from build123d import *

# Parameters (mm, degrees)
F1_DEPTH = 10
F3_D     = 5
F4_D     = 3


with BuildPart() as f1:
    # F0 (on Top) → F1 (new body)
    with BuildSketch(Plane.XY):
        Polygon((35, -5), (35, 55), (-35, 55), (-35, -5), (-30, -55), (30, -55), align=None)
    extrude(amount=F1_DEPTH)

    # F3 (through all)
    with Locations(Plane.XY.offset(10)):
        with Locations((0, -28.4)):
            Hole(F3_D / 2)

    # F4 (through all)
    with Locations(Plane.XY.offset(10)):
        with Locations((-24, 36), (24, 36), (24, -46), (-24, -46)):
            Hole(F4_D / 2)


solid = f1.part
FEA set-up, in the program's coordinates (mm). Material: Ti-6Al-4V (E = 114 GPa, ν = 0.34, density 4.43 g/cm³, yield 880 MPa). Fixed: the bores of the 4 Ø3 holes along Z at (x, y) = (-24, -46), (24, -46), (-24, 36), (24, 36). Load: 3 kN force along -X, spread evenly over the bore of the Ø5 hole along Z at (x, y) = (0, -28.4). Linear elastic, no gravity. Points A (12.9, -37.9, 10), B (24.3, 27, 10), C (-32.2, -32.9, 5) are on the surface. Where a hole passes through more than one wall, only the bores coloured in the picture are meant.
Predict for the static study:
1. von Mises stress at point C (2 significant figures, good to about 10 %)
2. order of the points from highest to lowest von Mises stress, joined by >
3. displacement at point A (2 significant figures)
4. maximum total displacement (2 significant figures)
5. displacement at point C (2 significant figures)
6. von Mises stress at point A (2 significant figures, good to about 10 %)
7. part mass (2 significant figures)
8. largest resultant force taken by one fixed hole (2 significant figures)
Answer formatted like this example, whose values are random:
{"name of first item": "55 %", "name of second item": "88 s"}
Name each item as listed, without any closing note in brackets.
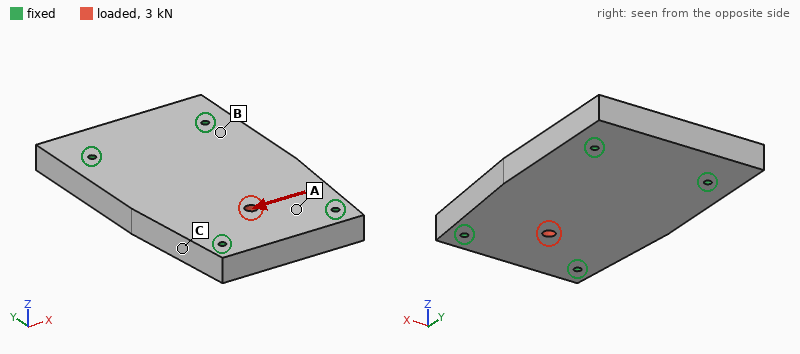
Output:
{"von Mises stress at point C": "4.9 MPa", "order of the points from highest to lowest von Mises stress, joined by >": "A > C > B", "displacement at point A": "1.3 µm", "maximum total displacement": "3.3 µm", "displacement at point C": "1.5 µm", "von Mises stress at point A": "8.8 MPa", "part mass": "330 g", "largest resultant force taken by one fixed hole": "1.2 kN"}
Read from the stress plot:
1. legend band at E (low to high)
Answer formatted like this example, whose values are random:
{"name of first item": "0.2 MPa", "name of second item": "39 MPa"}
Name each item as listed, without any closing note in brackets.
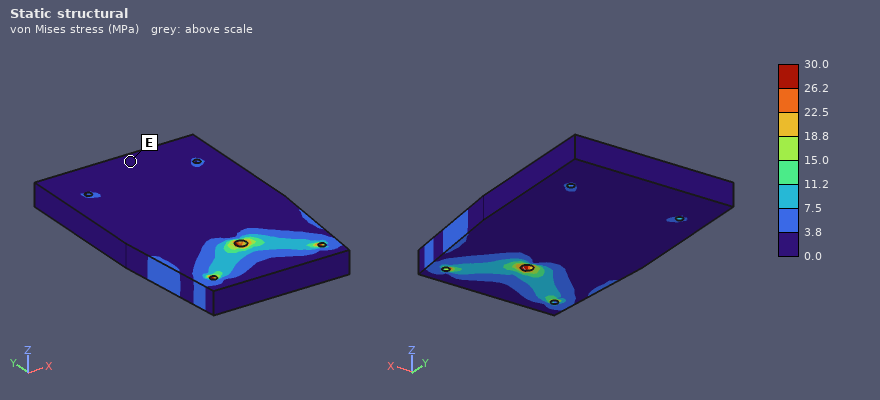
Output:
{"legend band at E": "0.0 to 3.8 MPa"}
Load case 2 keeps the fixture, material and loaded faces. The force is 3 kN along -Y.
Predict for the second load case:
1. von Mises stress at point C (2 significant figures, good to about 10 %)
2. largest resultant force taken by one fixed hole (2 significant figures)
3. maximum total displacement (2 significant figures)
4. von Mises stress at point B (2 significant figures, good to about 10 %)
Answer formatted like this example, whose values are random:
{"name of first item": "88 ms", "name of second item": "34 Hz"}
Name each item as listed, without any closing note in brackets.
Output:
{"von Mises stress at point C": "2.3 MPa", "largest resultant force taken by one fixed hole": "980 N", "maximum total displacement": "2.9 µm", "von Mises stress at point B": "3.0 MPa"}
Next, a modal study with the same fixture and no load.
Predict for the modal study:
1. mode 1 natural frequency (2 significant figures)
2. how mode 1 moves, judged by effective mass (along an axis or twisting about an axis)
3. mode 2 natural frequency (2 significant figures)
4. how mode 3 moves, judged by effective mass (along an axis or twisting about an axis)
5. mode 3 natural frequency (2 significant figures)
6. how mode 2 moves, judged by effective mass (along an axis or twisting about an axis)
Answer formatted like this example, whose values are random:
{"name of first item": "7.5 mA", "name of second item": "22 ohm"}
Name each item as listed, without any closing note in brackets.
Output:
{"mode 1 natural frequency": "5500 Hz", "how mode 1 moves, judged by effective mass": "along Z", "mode 2 natural frequency": "7800 Hz", "how mode 3 moves, judged by effective mass": "along Z", "mode 3 natural frequency": "11 kHz", "how mode 2 moves, judged by effective mass": "twisting about Y"}
